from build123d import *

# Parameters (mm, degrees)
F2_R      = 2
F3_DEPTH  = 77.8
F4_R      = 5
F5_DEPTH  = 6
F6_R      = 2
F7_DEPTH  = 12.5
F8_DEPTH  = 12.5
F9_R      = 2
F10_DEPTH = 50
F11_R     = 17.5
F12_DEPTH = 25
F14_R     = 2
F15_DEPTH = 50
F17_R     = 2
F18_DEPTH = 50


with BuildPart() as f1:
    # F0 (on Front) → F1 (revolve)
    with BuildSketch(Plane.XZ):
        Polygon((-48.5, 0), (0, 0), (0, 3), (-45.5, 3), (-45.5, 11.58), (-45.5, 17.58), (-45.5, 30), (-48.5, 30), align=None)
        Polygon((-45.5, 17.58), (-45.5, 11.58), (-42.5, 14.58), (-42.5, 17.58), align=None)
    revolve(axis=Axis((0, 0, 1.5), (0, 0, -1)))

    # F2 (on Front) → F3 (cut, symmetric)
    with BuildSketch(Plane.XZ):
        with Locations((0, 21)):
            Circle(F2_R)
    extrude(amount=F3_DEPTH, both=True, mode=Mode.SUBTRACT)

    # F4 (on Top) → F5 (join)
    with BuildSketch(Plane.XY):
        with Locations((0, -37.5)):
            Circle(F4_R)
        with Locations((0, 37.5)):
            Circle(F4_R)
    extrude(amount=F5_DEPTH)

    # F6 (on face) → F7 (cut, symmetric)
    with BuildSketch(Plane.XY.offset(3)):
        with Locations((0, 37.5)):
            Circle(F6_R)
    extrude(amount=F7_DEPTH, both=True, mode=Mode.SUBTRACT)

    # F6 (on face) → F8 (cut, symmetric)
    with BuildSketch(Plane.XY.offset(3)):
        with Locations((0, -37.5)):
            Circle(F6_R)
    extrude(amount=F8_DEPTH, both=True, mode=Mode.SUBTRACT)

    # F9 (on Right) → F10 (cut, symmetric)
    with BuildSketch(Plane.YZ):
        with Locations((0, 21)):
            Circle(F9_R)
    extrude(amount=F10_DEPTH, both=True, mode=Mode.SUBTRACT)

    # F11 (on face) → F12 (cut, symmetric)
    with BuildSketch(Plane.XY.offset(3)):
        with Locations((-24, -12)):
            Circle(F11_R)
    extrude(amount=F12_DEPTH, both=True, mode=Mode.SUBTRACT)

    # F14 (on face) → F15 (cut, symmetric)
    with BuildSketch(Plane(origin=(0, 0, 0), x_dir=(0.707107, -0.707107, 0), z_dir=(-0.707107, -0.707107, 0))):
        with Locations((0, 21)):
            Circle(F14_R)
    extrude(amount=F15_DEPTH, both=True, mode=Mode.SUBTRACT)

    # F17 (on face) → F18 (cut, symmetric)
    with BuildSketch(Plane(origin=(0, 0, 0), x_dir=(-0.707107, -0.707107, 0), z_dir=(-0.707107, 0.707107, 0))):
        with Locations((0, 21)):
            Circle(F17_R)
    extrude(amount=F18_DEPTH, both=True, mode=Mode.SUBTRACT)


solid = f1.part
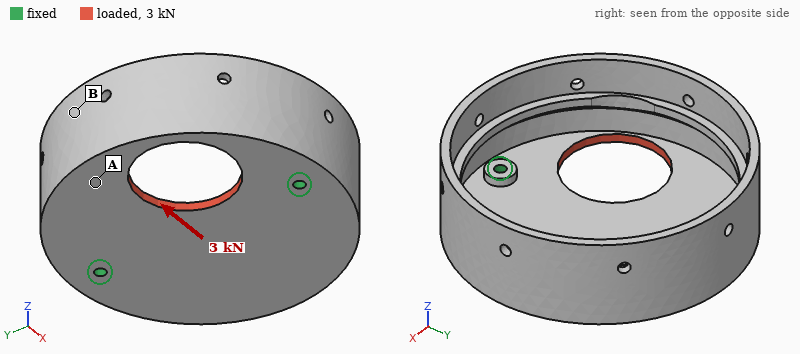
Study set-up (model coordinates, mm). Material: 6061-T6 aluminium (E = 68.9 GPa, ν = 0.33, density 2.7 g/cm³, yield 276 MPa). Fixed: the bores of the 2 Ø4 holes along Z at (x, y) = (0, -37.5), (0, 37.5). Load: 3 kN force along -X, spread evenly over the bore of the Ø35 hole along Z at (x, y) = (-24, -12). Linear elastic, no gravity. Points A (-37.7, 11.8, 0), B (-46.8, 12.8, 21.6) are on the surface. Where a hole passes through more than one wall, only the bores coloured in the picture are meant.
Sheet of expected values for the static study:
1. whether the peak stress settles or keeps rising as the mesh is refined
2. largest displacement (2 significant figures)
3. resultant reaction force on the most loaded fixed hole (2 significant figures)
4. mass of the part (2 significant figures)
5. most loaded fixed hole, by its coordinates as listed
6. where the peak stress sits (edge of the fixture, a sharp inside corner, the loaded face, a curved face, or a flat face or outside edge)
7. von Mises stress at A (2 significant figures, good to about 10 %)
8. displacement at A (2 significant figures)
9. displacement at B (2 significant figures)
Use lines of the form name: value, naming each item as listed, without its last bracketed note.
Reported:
whether the peak stress settles or keeps rising as the mesh is refined: keeps rising
largest displacement: 38 µm
resultant reaction force on the most loaded fixed hole: 2.0 kN
mass of the part: 130 g
most loaded fixed hole, by its coordinates as listed: (0, -37.5)
where the peak stress sits: edge of the fixture
von Mises stress at A: 12 MPa
displacement at A: 19 µm
displacement at B: 20 µm
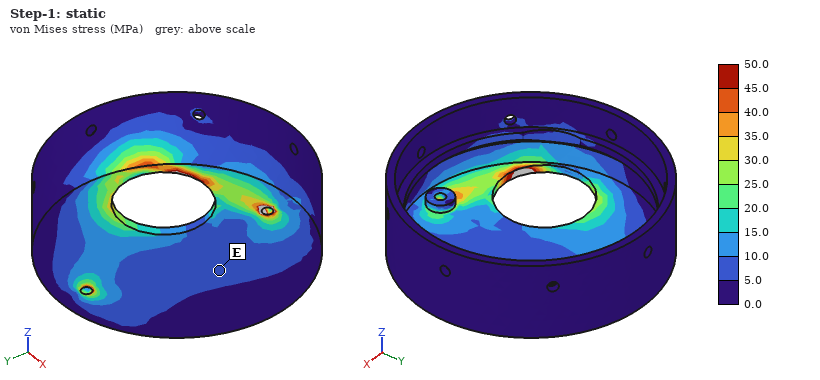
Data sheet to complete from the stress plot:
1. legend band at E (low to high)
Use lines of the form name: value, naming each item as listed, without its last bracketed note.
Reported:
legend band at E: 5.0 to 10.0 MPa
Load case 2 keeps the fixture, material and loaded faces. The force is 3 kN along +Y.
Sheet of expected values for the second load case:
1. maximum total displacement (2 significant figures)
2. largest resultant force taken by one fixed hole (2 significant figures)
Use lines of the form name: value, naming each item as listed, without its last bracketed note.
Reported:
maximum total displacement: 51 µm
largest resultant force taken by one fixed hole: 1.8 kN
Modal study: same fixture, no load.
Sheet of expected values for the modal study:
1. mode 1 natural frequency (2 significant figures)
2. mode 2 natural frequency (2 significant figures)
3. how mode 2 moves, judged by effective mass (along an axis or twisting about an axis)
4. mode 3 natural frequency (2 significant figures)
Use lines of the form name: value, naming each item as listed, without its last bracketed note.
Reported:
mode 1 natural frequency: 910 Hz
mode 2 natural frequency: 1800 Hz
how mode 2 moves, judged by effective mass: along Z
mode 3 natural frequency: 2100 Hz
